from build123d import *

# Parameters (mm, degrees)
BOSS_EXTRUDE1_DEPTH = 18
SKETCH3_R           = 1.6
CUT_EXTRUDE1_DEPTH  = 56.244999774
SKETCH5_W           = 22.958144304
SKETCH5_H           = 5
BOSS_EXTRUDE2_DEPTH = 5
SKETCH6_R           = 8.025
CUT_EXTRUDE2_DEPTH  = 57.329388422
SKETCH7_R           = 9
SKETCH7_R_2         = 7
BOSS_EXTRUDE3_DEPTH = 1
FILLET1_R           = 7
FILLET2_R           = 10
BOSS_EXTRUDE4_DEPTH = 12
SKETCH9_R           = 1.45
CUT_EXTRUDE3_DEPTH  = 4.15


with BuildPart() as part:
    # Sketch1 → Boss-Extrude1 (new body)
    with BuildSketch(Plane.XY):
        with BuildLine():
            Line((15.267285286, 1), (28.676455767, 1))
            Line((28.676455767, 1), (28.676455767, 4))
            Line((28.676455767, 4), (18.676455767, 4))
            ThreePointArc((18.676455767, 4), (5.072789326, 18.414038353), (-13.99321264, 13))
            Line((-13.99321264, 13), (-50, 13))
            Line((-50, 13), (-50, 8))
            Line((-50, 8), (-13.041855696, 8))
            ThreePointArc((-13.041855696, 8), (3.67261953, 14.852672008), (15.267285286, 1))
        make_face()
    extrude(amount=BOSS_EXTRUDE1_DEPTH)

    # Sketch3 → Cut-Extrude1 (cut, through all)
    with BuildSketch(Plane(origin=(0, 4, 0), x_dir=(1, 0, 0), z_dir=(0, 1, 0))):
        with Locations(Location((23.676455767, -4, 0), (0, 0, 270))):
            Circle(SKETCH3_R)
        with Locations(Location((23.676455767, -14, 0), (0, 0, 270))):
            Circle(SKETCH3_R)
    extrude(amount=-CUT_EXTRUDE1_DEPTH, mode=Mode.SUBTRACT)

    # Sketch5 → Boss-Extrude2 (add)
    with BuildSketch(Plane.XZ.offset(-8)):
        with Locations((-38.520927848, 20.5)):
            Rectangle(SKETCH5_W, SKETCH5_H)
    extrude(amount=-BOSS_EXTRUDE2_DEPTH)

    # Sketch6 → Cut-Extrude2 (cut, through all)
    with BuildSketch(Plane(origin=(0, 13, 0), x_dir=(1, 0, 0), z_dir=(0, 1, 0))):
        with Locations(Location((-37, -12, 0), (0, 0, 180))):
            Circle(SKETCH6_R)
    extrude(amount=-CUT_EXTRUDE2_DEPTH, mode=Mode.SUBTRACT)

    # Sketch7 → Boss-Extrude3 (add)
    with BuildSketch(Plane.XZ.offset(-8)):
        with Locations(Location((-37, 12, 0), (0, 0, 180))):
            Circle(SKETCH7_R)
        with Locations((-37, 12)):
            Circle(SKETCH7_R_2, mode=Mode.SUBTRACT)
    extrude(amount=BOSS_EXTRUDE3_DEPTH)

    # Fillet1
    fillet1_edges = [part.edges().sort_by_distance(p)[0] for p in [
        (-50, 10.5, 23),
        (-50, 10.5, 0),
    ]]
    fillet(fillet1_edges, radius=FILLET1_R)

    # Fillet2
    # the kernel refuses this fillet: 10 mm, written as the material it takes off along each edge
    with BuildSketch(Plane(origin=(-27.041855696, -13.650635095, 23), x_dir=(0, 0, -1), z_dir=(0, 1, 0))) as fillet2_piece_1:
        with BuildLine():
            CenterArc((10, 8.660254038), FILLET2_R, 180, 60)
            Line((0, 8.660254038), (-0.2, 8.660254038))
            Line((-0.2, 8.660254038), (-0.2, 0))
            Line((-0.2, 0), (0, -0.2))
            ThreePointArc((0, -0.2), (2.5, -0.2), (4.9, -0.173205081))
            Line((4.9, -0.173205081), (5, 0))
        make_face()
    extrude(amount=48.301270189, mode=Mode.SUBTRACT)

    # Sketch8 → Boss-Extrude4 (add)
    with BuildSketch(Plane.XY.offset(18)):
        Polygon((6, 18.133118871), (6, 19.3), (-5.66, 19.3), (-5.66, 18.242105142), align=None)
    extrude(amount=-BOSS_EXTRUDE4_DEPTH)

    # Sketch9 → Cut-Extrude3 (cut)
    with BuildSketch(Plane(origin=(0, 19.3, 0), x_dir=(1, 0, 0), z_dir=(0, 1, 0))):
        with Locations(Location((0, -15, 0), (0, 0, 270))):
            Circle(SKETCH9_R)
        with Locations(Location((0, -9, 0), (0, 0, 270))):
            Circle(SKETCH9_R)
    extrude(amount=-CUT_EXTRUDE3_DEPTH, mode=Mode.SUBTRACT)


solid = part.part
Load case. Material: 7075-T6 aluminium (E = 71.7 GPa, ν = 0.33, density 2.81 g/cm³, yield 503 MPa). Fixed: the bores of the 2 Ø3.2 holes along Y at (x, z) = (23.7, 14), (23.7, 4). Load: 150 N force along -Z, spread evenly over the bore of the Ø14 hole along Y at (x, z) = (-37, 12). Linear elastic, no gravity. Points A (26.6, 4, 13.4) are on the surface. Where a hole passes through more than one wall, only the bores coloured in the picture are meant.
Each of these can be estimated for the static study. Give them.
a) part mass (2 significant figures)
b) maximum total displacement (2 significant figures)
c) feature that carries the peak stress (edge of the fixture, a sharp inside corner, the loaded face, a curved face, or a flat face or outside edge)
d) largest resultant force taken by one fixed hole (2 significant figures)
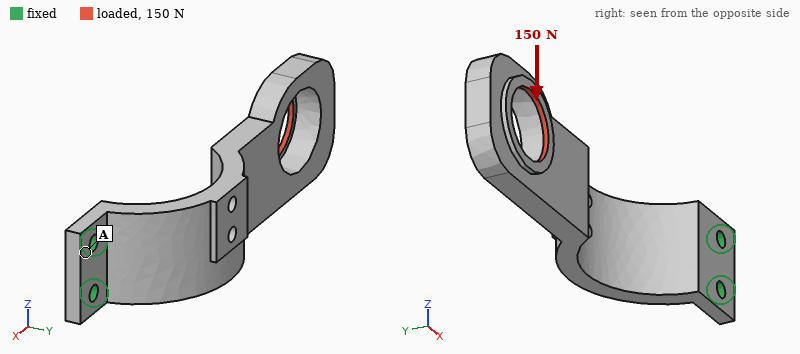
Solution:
17 g
0.76 mm
a curved face
780 N
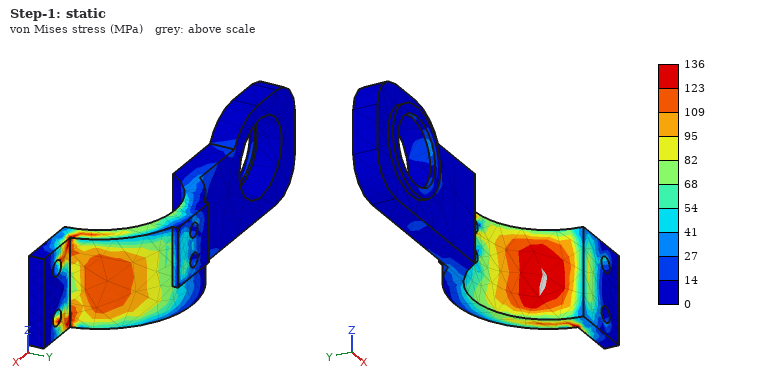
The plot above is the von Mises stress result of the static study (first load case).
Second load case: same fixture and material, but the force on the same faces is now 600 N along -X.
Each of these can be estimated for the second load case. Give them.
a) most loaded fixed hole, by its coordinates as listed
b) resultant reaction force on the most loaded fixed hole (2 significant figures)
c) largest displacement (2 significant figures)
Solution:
(23.7, 14)
460 N
0.91 mm
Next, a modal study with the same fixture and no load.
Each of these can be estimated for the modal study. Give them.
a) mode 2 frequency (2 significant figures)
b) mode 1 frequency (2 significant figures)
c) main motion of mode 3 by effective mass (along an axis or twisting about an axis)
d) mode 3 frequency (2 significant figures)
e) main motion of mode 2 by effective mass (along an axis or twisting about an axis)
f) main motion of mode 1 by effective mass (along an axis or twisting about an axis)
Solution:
990 Hz
460 Hz
along X
2300 Hz
along Z
along Y
